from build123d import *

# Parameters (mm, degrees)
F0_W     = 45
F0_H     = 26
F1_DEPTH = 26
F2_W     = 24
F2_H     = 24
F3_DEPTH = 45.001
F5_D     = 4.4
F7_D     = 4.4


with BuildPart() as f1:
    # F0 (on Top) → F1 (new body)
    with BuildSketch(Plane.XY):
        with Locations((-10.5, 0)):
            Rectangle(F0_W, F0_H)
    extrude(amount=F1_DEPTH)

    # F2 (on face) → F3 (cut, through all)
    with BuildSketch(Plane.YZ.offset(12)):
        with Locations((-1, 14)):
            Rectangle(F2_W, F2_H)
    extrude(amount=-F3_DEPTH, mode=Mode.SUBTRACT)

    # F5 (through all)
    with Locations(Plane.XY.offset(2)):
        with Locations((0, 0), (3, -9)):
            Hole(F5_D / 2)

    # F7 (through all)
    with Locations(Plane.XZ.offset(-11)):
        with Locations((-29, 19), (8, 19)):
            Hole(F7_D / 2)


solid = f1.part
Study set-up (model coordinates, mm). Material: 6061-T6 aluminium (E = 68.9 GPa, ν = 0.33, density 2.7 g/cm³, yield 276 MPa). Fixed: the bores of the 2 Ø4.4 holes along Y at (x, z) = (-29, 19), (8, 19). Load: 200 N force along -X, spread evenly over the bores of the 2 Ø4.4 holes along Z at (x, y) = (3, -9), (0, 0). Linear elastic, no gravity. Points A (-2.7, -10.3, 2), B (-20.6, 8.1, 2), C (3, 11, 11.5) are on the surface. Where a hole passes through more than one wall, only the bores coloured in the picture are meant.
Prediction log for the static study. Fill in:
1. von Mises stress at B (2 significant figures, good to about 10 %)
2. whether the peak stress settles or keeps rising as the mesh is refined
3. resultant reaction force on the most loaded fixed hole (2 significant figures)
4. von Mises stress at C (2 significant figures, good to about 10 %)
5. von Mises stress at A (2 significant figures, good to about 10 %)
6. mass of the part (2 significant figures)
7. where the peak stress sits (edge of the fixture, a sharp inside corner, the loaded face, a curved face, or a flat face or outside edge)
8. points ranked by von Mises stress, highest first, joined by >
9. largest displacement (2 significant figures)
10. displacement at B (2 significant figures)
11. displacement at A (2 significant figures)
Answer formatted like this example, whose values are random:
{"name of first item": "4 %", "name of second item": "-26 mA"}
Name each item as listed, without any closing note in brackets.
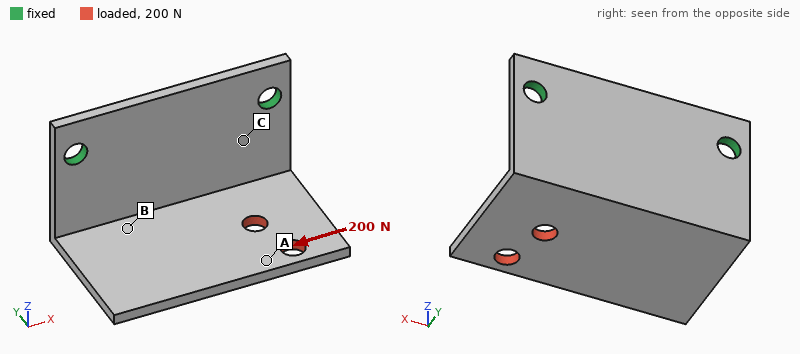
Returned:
{"von Mises stress at B": "29 MPa", "whether the peak stress settles or keeps rising as the mesh is refined": "keeps rising", "resultant reaction force on the most loaded fixed hole": "160 N", "von Mises stress at C": "45 MPa", "von Mises stress at A": "10 MPa", "mass of the part": "12 g", "where the peak stress sits": "edge of the fixture", "points ranked by von Mises stress, highest first, joined by >": "C > B > A", "largest displacement": "0.20 mm", "displacement at B": "0.056 mm", "displacement at A": "0.13 mm"}
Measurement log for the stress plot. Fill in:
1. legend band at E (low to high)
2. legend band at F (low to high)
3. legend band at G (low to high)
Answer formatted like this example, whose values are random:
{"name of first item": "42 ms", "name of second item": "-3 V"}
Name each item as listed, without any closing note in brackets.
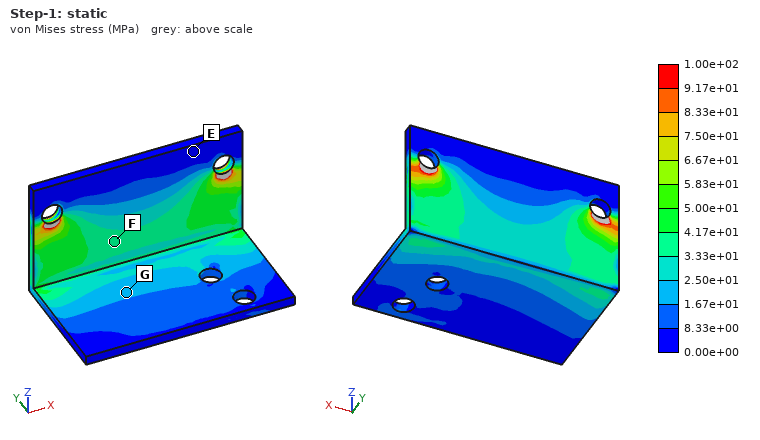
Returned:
{"legend band at E": "0.00e+00 to 8.33e+00 MPa", "legend band at F": "3.33e+01 to 4.17e+01 MPa", "legend band at G": "1.67e+01 to 2.50e+01 MPa"}
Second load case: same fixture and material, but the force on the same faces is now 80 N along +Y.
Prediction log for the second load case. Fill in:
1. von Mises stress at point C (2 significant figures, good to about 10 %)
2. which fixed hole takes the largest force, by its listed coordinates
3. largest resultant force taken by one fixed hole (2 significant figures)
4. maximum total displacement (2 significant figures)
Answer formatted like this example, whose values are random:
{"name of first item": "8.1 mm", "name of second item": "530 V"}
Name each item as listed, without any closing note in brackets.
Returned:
{"von Mises stress at point C": "38 MPa", "which fixed hole takes the largest force, by its listed coordinates": "(8, 19)", "largest resultant force taken by one fixed hole": "67 N", "maximum total displacement": "0.23 mm"}
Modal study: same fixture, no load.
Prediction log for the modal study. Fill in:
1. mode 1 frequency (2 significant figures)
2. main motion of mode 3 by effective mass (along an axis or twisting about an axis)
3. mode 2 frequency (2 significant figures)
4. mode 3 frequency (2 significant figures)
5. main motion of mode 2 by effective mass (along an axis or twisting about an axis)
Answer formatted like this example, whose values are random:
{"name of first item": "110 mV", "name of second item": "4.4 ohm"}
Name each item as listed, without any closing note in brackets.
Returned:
{"mode 1 frequency": "1200 Hz", "main motion of mode 3 by effective mass": "along Y", "mode 2 frequency": "2400 Hz", "mode 3 frequency": "3200 Hz", "main motion of mode 2 by effective mass": "along X"}
